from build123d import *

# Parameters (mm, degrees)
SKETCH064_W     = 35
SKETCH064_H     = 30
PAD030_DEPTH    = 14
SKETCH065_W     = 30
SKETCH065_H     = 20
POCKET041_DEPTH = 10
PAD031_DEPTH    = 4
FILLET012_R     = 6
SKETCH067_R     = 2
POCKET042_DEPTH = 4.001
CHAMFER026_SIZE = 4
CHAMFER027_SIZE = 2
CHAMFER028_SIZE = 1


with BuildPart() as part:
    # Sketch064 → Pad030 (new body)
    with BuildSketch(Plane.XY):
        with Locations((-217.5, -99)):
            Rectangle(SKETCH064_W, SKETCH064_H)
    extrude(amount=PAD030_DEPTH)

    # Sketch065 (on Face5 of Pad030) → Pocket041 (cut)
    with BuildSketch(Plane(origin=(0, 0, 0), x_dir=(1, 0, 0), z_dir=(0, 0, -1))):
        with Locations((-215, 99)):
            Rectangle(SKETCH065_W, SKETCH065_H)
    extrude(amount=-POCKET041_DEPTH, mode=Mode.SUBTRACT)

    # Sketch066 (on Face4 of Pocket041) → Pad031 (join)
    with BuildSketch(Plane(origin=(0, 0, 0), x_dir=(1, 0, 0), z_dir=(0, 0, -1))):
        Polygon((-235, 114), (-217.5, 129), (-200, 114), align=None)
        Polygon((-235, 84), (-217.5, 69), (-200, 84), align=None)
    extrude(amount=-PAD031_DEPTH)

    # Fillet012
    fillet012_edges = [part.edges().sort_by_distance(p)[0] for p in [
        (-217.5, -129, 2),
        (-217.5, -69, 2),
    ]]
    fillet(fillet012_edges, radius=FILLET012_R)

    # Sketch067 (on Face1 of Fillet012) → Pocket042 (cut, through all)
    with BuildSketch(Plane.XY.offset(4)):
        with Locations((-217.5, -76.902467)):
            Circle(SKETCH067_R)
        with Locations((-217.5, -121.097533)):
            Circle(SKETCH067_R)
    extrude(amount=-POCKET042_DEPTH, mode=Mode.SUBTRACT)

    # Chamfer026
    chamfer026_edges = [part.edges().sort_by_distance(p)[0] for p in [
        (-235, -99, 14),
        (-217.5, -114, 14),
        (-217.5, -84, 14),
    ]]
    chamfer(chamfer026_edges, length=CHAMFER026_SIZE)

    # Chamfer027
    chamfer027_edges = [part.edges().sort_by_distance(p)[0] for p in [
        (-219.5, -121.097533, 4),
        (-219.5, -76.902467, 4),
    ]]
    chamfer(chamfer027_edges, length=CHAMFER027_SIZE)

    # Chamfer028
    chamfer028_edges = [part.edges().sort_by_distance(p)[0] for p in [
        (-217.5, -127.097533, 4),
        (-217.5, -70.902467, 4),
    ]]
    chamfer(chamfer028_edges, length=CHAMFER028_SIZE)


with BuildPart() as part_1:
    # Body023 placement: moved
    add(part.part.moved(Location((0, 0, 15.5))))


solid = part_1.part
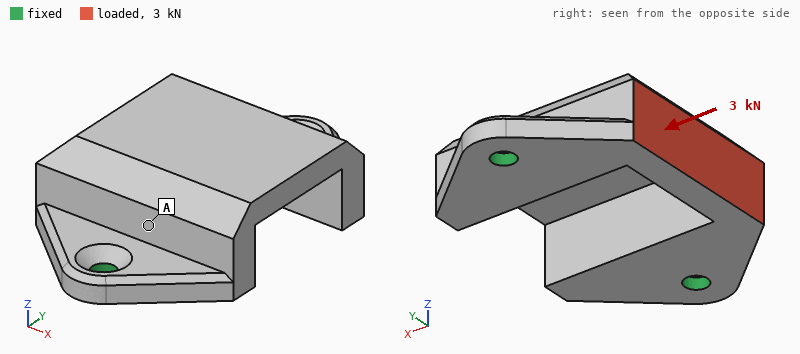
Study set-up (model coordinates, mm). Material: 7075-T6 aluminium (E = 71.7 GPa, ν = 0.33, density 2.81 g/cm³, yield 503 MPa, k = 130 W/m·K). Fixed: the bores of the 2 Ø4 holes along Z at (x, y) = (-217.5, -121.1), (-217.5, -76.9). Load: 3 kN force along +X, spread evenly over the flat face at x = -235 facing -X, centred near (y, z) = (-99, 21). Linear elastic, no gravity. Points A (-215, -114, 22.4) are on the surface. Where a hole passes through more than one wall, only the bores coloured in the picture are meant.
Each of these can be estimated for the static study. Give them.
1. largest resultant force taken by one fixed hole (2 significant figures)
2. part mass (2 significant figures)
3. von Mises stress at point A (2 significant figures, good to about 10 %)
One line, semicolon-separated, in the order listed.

1.7 kN; 28 g; 32 MPa
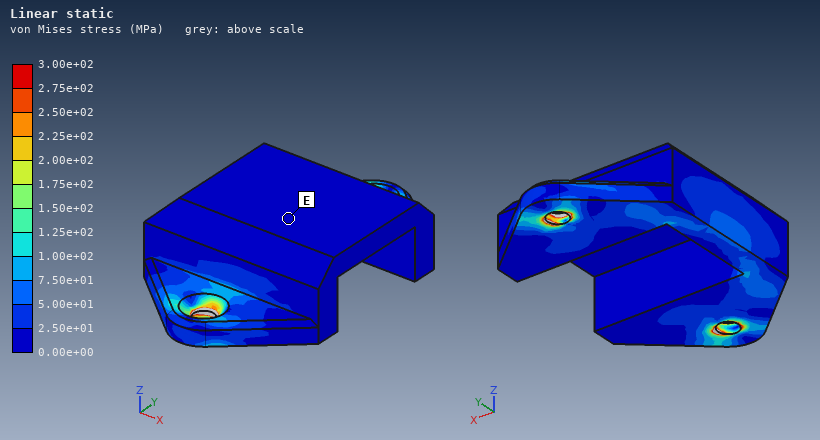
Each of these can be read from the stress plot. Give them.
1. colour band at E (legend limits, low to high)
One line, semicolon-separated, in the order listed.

0.00e+00 to 2.50e+01 MPa
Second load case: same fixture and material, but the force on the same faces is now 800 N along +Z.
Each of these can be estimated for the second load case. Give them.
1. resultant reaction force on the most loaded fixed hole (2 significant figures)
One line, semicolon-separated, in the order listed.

470 N
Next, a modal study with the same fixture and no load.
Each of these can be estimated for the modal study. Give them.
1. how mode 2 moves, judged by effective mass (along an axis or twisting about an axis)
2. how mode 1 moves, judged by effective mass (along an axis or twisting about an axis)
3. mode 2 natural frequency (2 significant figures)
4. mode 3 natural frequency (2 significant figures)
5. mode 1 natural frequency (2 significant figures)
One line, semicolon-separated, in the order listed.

along Z; along X; 9700 Hz; 11 kHz; 3200 Hz
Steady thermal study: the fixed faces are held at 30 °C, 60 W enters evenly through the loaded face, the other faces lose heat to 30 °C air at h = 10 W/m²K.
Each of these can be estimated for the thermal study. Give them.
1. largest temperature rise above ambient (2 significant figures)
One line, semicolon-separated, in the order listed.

70 K
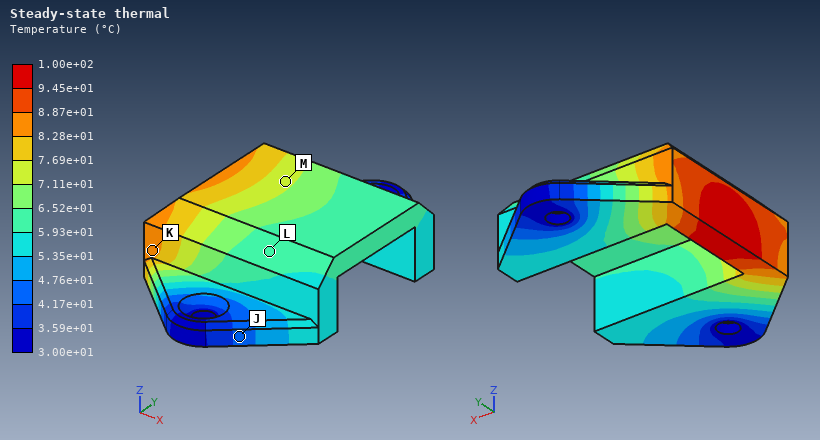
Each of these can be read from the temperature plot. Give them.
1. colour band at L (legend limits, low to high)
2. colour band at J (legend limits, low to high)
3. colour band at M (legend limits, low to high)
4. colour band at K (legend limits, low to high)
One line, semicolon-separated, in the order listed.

5.93e+01 to 6.52e+01 °C; 4.17e+01 to 4.76e+01 °C; 7.11e+01 to 7.69e+01 °C; 8.28e+01 to 8.87e+01 °C
